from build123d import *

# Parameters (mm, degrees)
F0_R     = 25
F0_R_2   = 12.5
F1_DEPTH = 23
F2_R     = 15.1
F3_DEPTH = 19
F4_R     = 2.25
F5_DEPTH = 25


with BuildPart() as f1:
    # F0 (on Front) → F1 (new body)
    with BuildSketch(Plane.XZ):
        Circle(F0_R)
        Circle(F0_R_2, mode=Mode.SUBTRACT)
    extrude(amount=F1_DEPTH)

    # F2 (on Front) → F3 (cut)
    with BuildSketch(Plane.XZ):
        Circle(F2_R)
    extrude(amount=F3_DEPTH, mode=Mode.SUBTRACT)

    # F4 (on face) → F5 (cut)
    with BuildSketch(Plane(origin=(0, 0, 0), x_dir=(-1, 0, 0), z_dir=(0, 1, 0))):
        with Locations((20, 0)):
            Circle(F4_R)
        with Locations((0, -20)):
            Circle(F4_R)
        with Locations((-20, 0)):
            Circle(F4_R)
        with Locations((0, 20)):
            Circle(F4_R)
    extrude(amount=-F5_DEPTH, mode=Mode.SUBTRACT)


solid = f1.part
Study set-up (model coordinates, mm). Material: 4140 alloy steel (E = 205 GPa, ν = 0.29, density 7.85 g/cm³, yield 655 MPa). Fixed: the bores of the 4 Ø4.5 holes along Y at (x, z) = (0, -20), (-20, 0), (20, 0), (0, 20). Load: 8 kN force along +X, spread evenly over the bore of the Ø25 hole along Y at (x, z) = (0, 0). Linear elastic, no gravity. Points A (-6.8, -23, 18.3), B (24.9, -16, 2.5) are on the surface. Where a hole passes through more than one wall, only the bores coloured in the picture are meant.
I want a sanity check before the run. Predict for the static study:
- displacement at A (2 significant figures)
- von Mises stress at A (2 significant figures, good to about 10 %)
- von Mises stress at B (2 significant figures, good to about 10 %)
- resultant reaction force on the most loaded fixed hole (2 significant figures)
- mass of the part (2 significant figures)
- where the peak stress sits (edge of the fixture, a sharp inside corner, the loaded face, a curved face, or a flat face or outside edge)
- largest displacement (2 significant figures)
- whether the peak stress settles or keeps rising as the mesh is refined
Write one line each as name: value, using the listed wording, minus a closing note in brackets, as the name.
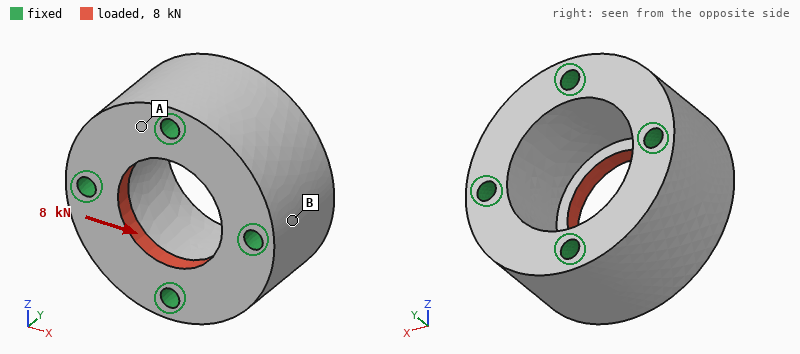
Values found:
displacement at A: 0.74 µm
von Mises stress at A: 16 MPa
von Mises stress at B: 7.9 MPa
resultant reaction force on the most loaded fixed hole: 2.2 kN
mass of the part: 220 g
where the peak stress sits: edge of the fixture
largest displacement: 2.3 µm
whether the peak stress settles or keeps rising as the mesh is refined: keeps rising
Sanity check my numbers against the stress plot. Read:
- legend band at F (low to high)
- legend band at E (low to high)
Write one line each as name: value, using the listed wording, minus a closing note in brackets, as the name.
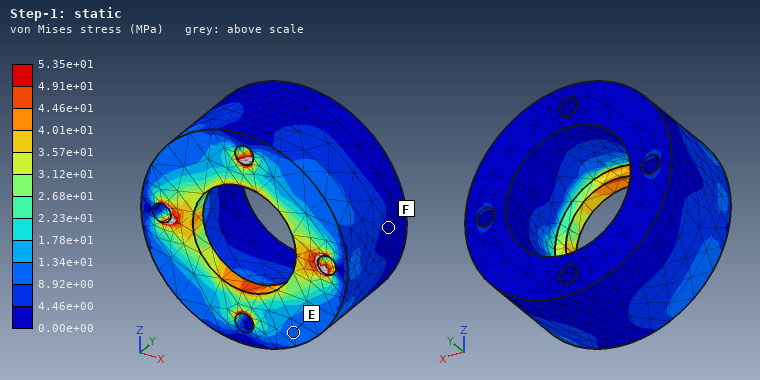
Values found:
legend band at F: 0.00e+00 to 4.46e+00 MPa
legend band at E: 8.92e+00 to 1.34e+01 MPa
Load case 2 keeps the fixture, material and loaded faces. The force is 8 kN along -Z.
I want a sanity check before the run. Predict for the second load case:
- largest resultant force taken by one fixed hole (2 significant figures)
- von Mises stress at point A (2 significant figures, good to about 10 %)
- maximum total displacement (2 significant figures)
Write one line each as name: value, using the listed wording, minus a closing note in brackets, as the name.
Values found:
largest resultant force taken by one fixed hole: 2.2 kN
von Mises stress at point A: 20 MPa
maximum total displacement: 2.3 µm
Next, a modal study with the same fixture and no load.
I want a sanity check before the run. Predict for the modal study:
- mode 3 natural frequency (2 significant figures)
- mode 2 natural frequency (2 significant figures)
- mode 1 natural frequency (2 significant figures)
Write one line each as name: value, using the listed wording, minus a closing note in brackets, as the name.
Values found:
mode 3 natural frequency: 44 kHz
mode 2 natural frequency: 44 kHz
mode 1 natural frequency: 43 kHz
